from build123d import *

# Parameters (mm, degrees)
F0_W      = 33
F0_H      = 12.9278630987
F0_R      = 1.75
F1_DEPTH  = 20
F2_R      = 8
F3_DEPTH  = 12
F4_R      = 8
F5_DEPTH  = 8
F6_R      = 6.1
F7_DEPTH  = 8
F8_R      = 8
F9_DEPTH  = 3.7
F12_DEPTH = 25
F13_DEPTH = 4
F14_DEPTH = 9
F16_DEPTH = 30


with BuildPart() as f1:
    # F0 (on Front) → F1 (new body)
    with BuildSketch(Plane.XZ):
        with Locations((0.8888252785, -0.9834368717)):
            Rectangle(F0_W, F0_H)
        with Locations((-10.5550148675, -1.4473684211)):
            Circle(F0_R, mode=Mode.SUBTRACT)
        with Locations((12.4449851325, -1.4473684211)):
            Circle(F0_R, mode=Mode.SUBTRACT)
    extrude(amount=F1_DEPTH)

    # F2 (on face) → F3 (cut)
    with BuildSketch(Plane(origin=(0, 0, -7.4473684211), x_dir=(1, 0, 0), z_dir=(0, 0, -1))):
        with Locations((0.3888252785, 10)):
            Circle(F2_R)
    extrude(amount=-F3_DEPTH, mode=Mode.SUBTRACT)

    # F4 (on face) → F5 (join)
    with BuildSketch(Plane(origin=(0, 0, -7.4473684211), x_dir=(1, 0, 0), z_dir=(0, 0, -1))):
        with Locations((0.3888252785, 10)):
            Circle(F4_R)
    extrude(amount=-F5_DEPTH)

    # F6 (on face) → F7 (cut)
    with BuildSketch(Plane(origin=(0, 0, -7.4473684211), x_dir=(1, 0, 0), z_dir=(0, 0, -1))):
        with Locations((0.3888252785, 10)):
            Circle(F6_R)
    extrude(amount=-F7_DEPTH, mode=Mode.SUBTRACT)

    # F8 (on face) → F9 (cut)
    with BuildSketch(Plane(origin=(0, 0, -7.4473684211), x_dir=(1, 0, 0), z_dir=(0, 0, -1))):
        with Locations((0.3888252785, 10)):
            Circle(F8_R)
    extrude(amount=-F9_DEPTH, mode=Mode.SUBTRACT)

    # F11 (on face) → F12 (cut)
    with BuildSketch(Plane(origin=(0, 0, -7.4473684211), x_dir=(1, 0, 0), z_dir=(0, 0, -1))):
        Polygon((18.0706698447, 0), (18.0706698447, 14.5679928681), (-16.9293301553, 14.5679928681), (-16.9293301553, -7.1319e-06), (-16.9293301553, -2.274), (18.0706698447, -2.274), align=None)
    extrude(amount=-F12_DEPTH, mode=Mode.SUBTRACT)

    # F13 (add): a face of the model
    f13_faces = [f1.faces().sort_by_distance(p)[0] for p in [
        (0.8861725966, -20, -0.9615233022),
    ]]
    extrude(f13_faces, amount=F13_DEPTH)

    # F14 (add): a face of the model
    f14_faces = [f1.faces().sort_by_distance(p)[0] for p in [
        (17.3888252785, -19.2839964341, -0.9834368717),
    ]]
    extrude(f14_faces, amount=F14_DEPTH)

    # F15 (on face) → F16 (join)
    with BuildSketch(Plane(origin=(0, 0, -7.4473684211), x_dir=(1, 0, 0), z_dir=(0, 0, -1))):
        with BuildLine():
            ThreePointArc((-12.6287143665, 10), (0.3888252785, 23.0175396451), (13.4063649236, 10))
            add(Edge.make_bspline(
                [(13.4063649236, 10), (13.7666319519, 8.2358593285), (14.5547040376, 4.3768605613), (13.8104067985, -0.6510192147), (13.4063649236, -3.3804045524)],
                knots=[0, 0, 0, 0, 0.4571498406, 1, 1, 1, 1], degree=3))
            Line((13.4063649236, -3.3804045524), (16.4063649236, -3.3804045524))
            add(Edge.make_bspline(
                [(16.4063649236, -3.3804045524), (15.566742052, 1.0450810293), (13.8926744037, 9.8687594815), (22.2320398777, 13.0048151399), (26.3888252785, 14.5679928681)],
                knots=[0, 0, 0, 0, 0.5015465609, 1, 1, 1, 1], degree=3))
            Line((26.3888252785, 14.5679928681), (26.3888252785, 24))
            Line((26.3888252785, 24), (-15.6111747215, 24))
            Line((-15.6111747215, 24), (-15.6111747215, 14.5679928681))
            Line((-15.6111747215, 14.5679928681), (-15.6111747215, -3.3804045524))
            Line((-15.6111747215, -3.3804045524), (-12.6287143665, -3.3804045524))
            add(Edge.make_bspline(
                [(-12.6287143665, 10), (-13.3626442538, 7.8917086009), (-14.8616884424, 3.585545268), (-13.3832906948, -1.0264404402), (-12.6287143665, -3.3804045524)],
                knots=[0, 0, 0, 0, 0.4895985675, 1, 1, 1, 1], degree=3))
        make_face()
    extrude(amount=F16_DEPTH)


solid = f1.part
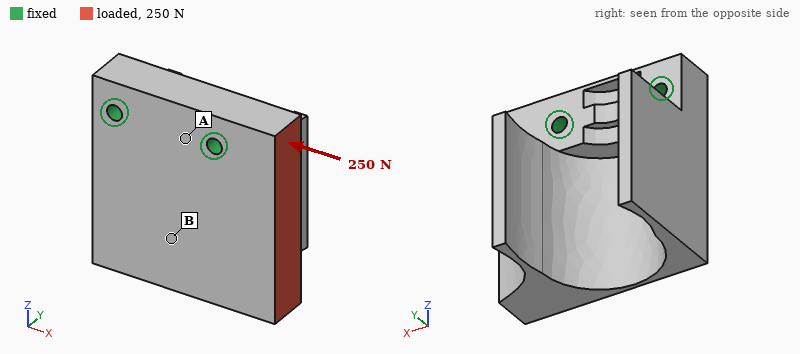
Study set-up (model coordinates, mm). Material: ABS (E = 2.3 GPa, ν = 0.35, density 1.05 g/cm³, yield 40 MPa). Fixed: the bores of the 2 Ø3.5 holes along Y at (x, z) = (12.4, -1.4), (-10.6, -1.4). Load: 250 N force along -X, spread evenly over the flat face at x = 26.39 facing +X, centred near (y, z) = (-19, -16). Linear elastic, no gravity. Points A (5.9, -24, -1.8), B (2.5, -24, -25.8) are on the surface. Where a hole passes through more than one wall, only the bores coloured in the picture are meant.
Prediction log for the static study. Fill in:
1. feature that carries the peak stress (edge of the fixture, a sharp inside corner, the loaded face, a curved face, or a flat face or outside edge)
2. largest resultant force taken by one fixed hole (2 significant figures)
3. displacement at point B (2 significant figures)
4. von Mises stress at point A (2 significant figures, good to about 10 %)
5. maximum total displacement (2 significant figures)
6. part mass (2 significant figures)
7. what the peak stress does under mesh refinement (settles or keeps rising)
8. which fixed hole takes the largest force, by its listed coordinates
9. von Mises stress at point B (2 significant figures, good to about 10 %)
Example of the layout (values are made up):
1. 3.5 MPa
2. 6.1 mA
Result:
1. edge of the fixture
2. 230 N
3. 0.062 mm
4. 1.1 MPa
5. 0.18 mm
6. 16 g
7. keeps rising
8. (12.4, -1.4)
9. 3.4 MPa
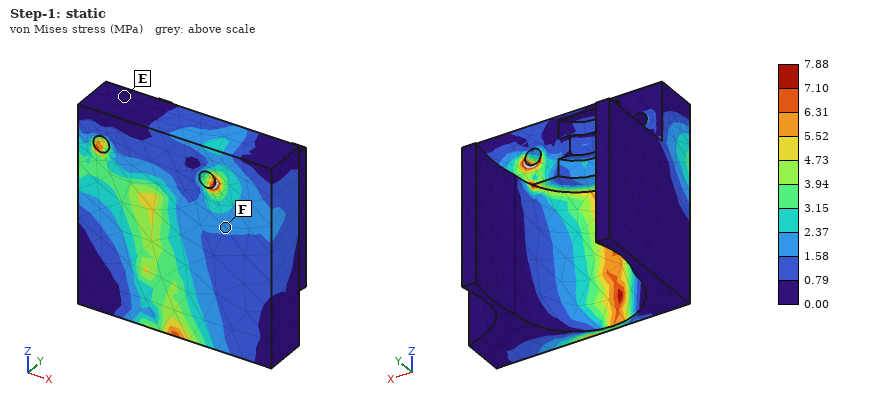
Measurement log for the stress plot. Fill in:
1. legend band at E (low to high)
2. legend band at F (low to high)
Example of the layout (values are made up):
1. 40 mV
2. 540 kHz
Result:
1. 0.00 to 0.79 MPa
2. 1.58 to 2.37 MPa
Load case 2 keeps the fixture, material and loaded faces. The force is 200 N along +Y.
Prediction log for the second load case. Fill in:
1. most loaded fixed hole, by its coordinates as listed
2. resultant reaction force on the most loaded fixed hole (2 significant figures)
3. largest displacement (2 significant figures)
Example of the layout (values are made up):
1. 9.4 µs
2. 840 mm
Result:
1. (12.4, -1.4)
2. 230 N
3. 0.56 mm
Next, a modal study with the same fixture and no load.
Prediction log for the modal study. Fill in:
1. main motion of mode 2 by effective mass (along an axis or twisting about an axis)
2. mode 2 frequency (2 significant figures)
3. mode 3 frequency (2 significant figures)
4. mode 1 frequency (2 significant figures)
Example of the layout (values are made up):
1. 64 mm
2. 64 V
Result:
1. along Y
2. 1300 Hz
3. 1600 Hz
4. 1200 Hz
